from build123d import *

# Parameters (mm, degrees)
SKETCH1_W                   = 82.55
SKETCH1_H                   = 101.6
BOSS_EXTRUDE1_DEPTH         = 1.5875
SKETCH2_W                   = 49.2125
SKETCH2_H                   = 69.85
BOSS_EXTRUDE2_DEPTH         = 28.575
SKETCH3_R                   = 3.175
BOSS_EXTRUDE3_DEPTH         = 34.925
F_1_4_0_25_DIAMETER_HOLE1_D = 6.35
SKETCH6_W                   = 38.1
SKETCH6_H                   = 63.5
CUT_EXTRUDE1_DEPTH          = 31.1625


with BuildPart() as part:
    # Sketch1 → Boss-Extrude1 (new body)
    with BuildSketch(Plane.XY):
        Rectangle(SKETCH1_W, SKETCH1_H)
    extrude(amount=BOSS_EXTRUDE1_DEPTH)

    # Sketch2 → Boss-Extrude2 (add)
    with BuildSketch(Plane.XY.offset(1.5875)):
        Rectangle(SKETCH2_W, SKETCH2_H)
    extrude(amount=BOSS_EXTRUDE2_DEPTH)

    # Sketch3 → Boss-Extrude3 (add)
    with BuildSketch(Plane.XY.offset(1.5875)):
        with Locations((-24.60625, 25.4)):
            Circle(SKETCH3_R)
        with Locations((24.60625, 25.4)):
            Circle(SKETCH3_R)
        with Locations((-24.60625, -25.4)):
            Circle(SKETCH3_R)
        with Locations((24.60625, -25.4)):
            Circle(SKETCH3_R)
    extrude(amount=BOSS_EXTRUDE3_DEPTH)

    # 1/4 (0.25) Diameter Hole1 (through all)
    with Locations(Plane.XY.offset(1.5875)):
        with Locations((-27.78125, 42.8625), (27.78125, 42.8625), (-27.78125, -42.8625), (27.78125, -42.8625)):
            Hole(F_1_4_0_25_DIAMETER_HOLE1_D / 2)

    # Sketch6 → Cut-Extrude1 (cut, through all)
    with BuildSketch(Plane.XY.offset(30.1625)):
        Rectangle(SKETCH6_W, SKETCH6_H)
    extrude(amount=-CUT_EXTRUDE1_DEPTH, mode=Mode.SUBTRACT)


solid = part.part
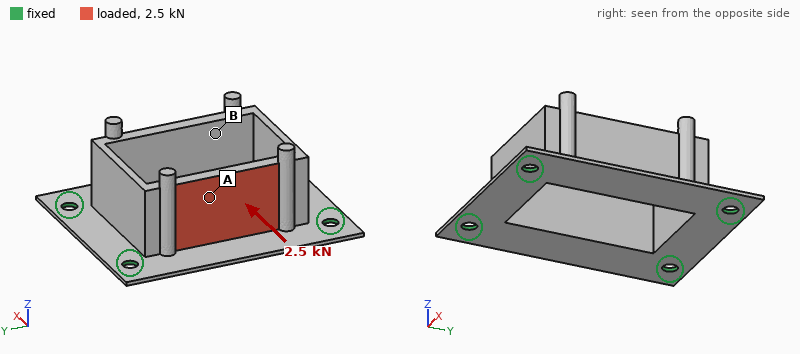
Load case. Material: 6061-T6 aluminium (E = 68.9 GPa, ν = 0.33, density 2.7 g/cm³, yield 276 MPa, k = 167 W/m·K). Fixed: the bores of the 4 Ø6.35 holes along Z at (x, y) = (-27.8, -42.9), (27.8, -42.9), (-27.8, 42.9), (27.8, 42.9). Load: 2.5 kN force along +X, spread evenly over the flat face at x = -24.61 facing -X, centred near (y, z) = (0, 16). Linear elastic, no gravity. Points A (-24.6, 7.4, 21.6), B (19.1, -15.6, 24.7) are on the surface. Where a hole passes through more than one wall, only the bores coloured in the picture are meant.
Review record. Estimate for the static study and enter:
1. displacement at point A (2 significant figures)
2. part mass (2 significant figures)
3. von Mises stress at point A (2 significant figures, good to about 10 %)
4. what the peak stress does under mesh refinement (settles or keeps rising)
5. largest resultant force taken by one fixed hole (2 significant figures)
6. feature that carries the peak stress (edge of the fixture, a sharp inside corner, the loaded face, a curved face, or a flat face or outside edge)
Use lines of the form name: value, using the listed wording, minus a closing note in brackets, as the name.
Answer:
displacement at point A: 0.19 mm
part mass: 110 g
von Mises stress at point A: 58 MPa
what the peak stress does under mesh refinement: keeps rising
largest resultant force taken by one fixed hole: 810 N
feature that carries the peak stress: edge of the fixture
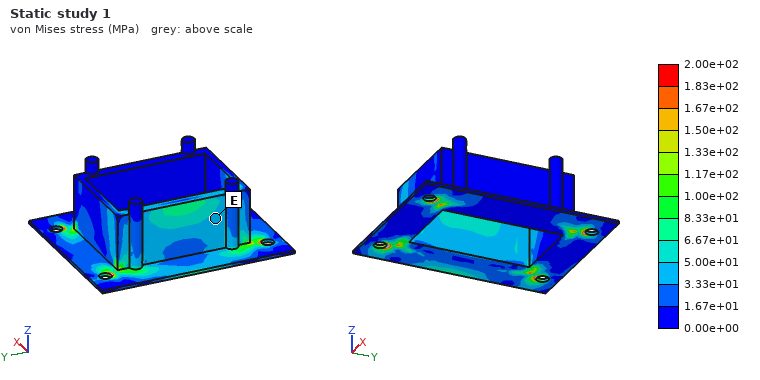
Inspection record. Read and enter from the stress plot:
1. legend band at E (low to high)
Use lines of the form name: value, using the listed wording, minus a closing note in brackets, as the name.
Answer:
legend band at E: 3.33e+01 to 5.00e+01 MPa
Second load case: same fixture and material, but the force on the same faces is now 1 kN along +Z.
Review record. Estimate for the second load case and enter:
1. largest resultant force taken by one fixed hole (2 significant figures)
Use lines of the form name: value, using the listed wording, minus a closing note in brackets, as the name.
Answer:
largest resultant force taken by one fixed hole: 590 N
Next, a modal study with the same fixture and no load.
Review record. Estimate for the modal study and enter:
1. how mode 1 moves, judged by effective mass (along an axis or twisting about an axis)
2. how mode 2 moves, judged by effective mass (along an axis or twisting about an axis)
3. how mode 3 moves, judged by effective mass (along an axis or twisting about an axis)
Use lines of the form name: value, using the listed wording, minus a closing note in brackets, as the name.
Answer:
how mode 1 moves, judged by effective mass: along X
how mode 2 moves, judged by effective mass: along Z
how mode 3 moves, judged by effective mass: along Y
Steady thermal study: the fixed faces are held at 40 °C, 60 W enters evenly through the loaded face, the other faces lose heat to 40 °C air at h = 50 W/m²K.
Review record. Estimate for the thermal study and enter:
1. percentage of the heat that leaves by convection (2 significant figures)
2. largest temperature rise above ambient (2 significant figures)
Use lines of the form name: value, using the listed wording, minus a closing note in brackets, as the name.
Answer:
percentage of the heat that leaves by convection: 36 %
largest temperature rise above ambient: 48 K
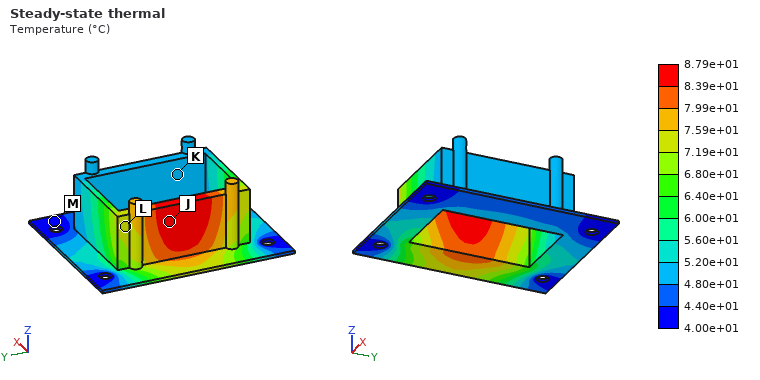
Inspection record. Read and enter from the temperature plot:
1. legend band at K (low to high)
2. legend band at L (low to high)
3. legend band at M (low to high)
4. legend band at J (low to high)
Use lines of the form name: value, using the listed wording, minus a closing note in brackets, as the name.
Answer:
legend band at K: 4.80e+01 to 5.20e+01 °C
legend band at L: 7.19e+01 to 7.59e+01 °C
legend band at M: 4.00e+01 to 4.40e+01 °C
legend band at J: 8.39e+01 to 8.79e+01 °C
